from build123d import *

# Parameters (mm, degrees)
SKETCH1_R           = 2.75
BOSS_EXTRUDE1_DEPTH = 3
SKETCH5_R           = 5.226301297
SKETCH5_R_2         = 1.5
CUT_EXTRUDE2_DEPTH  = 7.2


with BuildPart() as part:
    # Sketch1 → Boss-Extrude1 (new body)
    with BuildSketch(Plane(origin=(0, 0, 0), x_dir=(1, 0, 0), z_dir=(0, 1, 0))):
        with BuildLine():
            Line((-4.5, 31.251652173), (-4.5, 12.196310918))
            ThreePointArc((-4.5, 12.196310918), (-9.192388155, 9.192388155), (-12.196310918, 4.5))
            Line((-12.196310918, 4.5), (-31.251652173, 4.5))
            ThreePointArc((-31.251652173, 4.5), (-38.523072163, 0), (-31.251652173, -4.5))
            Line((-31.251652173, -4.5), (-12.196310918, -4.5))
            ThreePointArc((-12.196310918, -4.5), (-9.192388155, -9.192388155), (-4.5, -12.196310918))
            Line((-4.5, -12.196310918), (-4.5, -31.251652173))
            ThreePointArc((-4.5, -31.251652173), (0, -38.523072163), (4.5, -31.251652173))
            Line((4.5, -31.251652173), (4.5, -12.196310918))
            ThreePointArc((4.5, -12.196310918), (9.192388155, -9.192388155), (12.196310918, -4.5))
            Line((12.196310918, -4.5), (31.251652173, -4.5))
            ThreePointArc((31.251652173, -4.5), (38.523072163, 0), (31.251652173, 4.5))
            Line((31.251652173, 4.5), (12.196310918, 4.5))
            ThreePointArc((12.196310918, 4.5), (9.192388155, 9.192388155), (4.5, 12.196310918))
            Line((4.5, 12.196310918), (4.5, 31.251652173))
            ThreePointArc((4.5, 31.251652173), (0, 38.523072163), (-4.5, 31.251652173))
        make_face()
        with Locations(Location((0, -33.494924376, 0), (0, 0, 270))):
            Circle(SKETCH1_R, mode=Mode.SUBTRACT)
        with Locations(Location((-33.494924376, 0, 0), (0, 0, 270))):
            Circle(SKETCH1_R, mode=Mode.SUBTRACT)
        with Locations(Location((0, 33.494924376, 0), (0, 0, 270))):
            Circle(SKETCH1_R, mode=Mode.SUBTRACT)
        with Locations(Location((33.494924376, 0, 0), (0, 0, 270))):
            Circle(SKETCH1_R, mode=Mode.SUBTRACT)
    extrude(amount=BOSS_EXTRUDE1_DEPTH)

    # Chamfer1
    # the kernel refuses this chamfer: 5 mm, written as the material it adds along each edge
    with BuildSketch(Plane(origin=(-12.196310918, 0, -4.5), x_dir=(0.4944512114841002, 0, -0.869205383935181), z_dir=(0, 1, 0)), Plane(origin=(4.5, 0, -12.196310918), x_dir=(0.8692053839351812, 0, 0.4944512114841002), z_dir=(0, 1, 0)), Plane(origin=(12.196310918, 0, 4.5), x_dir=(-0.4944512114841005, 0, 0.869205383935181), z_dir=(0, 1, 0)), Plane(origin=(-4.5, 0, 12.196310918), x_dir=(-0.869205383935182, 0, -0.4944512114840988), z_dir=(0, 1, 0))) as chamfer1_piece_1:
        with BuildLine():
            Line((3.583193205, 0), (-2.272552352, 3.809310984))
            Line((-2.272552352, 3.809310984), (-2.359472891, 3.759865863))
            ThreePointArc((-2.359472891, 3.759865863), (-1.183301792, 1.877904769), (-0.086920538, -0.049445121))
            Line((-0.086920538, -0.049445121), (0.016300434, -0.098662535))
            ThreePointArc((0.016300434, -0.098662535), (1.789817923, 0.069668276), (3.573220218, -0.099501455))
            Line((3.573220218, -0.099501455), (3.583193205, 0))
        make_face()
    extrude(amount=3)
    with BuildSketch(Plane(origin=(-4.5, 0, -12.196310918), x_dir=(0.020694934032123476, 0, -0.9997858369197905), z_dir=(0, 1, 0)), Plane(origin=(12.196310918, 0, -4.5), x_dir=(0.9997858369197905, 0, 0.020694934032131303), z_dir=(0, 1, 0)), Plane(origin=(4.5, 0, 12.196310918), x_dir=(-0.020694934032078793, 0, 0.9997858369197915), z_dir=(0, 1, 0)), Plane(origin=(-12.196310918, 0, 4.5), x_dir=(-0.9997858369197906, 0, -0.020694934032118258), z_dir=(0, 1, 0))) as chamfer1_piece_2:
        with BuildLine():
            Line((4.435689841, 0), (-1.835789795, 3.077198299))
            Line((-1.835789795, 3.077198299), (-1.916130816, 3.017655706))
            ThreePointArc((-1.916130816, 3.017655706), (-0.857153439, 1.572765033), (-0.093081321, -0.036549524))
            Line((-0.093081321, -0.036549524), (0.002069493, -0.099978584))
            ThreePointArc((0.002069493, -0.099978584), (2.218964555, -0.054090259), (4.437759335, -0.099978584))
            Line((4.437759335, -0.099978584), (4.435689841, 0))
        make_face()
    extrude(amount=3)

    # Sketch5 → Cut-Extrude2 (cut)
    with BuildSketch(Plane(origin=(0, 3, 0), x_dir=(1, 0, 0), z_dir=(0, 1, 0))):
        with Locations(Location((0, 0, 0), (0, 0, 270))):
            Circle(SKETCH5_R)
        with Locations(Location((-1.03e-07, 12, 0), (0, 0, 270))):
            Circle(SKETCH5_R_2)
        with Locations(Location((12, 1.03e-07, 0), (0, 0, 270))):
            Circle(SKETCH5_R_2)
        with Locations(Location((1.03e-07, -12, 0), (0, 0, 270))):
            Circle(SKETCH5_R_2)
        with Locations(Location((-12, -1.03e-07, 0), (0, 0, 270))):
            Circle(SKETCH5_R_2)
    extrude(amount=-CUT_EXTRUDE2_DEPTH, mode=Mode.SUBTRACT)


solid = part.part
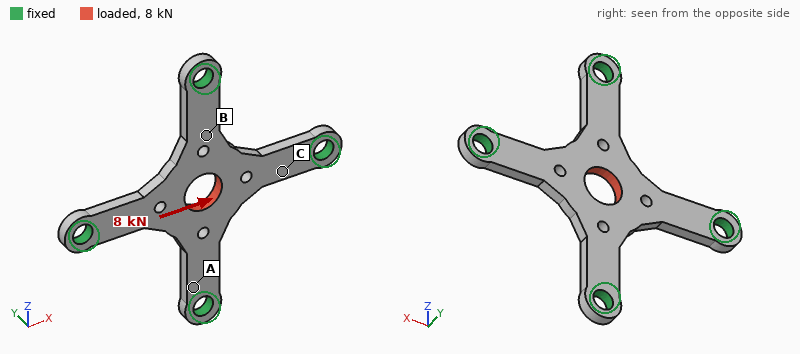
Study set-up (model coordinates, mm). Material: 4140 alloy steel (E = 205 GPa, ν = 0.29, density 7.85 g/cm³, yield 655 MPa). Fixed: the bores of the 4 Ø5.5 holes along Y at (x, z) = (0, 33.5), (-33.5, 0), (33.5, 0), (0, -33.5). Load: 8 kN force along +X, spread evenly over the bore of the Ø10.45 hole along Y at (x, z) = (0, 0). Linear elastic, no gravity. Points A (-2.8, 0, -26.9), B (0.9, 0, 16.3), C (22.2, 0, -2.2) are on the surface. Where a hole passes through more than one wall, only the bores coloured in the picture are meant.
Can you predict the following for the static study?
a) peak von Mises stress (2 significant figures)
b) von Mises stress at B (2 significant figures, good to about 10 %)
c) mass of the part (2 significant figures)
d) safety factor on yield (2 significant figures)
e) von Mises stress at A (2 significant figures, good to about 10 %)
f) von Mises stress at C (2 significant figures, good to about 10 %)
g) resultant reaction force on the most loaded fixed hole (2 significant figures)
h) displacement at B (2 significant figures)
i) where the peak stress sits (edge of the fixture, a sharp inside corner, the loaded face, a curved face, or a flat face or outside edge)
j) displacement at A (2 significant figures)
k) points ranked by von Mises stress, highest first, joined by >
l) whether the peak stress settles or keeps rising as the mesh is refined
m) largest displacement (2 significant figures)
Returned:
350 MPa
24 MPa
30 g
1.9
40 MPa
130 MPa
3.6 kN
12 µm
a curved face
2.9 µm
C > A > B
settles
19 µm
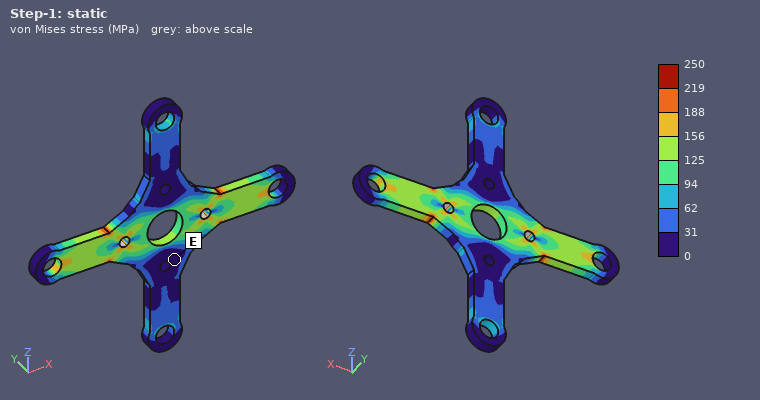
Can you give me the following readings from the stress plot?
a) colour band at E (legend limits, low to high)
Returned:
0 to 31 MPa
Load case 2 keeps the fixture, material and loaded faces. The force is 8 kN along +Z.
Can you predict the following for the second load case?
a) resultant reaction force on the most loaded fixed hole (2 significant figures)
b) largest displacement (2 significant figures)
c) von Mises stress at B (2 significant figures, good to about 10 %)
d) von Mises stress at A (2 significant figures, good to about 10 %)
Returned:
3.6 kN
19 µm
88 MPa
130 MPa
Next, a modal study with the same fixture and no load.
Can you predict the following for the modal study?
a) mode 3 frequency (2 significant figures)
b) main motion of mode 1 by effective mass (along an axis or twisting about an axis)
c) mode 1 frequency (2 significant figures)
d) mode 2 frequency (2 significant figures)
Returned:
10 kHz
along Y
4700 Hz
10 kHz
